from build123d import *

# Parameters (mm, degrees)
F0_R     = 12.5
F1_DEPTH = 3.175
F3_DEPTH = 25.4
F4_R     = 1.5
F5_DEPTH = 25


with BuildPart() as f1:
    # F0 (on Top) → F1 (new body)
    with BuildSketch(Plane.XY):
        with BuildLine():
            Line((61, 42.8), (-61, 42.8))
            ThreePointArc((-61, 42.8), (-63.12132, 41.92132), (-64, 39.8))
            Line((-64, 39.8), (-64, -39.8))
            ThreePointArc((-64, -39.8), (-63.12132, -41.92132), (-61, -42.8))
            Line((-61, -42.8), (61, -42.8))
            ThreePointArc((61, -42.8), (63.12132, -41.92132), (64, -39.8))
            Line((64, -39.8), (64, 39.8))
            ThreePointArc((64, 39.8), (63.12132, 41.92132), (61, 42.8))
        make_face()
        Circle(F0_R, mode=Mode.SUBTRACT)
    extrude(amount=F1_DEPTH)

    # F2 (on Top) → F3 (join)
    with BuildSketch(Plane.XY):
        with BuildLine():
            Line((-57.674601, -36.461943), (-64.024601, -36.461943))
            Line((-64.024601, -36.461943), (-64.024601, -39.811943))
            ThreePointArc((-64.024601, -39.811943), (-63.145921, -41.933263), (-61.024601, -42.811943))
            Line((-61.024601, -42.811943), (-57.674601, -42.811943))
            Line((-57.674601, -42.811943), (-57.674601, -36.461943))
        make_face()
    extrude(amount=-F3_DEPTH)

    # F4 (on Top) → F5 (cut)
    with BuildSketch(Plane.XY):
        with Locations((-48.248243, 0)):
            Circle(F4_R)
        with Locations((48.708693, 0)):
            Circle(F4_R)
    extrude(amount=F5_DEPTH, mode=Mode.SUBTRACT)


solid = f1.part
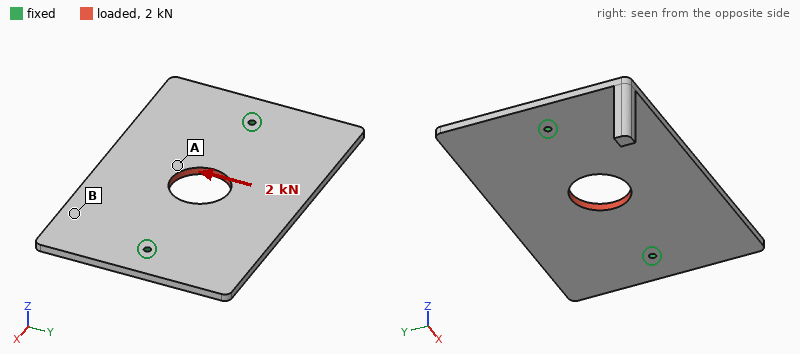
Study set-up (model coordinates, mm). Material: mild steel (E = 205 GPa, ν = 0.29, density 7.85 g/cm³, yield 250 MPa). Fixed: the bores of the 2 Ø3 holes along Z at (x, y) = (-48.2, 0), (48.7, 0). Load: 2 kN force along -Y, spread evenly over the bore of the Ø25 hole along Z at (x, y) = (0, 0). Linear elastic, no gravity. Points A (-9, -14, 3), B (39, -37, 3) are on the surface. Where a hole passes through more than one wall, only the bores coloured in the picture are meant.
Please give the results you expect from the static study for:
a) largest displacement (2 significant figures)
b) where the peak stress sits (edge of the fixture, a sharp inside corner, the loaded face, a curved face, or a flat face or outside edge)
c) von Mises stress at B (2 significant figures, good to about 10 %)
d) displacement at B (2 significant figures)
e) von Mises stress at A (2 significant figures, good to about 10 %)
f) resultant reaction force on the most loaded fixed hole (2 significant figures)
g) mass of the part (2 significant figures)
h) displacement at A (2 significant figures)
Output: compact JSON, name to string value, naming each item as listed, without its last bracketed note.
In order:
{"largest displacement": "4.3 µm", "where the peak stress sits": "edge of the fixture", "von Mises stress at B": "3.3 MPa", "displacement at B": "2.1 µm", "von Mises stress at A": "8.8 MPa", "resultant reaction force on the most loaded fixed hole": "1.0 kN", "mass of the part": "270 g", "displacement at A": "4.0 µm"}
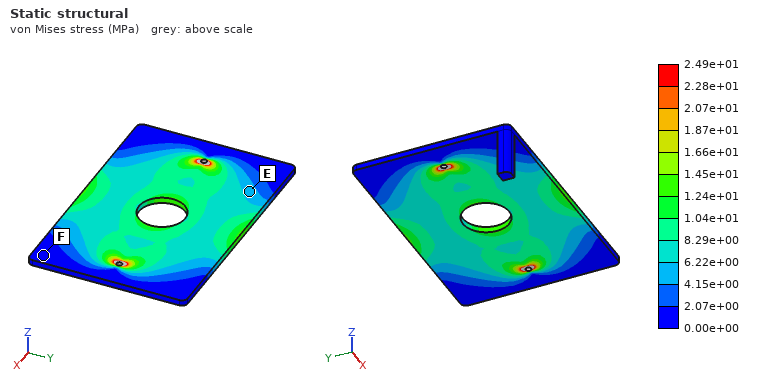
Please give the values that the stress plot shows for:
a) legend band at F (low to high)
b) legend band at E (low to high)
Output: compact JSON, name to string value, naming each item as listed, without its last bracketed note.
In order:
{"legend band at F": "0.00e+00 to 2.07e+00 MPa", "legend band at E": "4.15e+00 to 6.22e+00 MPa"}
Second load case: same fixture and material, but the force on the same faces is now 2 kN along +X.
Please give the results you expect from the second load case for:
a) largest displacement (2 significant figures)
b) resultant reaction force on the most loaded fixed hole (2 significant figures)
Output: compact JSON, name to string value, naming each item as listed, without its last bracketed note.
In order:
{"largest displacement": "2.5 µm", "resultant reaction force on the most loaded fixed hole": "1.0 kN"}
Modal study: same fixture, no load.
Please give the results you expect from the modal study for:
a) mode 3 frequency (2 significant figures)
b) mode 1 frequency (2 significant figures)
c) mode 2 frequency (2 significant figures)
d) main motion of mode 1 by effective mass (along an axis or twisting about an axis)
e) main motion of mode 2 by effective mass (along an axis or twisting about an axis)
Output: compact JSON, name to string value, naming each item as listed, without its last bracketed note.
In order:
{"mode 3 frequency": "1200 Hz", "mode 1 frequency": "750 Hz", "mode 2 frequency": "1000 Hz", "main motion of mode 1 by effective mass": "twisting about X", "main motion of mode 2 by effective mass": "along Z"}
